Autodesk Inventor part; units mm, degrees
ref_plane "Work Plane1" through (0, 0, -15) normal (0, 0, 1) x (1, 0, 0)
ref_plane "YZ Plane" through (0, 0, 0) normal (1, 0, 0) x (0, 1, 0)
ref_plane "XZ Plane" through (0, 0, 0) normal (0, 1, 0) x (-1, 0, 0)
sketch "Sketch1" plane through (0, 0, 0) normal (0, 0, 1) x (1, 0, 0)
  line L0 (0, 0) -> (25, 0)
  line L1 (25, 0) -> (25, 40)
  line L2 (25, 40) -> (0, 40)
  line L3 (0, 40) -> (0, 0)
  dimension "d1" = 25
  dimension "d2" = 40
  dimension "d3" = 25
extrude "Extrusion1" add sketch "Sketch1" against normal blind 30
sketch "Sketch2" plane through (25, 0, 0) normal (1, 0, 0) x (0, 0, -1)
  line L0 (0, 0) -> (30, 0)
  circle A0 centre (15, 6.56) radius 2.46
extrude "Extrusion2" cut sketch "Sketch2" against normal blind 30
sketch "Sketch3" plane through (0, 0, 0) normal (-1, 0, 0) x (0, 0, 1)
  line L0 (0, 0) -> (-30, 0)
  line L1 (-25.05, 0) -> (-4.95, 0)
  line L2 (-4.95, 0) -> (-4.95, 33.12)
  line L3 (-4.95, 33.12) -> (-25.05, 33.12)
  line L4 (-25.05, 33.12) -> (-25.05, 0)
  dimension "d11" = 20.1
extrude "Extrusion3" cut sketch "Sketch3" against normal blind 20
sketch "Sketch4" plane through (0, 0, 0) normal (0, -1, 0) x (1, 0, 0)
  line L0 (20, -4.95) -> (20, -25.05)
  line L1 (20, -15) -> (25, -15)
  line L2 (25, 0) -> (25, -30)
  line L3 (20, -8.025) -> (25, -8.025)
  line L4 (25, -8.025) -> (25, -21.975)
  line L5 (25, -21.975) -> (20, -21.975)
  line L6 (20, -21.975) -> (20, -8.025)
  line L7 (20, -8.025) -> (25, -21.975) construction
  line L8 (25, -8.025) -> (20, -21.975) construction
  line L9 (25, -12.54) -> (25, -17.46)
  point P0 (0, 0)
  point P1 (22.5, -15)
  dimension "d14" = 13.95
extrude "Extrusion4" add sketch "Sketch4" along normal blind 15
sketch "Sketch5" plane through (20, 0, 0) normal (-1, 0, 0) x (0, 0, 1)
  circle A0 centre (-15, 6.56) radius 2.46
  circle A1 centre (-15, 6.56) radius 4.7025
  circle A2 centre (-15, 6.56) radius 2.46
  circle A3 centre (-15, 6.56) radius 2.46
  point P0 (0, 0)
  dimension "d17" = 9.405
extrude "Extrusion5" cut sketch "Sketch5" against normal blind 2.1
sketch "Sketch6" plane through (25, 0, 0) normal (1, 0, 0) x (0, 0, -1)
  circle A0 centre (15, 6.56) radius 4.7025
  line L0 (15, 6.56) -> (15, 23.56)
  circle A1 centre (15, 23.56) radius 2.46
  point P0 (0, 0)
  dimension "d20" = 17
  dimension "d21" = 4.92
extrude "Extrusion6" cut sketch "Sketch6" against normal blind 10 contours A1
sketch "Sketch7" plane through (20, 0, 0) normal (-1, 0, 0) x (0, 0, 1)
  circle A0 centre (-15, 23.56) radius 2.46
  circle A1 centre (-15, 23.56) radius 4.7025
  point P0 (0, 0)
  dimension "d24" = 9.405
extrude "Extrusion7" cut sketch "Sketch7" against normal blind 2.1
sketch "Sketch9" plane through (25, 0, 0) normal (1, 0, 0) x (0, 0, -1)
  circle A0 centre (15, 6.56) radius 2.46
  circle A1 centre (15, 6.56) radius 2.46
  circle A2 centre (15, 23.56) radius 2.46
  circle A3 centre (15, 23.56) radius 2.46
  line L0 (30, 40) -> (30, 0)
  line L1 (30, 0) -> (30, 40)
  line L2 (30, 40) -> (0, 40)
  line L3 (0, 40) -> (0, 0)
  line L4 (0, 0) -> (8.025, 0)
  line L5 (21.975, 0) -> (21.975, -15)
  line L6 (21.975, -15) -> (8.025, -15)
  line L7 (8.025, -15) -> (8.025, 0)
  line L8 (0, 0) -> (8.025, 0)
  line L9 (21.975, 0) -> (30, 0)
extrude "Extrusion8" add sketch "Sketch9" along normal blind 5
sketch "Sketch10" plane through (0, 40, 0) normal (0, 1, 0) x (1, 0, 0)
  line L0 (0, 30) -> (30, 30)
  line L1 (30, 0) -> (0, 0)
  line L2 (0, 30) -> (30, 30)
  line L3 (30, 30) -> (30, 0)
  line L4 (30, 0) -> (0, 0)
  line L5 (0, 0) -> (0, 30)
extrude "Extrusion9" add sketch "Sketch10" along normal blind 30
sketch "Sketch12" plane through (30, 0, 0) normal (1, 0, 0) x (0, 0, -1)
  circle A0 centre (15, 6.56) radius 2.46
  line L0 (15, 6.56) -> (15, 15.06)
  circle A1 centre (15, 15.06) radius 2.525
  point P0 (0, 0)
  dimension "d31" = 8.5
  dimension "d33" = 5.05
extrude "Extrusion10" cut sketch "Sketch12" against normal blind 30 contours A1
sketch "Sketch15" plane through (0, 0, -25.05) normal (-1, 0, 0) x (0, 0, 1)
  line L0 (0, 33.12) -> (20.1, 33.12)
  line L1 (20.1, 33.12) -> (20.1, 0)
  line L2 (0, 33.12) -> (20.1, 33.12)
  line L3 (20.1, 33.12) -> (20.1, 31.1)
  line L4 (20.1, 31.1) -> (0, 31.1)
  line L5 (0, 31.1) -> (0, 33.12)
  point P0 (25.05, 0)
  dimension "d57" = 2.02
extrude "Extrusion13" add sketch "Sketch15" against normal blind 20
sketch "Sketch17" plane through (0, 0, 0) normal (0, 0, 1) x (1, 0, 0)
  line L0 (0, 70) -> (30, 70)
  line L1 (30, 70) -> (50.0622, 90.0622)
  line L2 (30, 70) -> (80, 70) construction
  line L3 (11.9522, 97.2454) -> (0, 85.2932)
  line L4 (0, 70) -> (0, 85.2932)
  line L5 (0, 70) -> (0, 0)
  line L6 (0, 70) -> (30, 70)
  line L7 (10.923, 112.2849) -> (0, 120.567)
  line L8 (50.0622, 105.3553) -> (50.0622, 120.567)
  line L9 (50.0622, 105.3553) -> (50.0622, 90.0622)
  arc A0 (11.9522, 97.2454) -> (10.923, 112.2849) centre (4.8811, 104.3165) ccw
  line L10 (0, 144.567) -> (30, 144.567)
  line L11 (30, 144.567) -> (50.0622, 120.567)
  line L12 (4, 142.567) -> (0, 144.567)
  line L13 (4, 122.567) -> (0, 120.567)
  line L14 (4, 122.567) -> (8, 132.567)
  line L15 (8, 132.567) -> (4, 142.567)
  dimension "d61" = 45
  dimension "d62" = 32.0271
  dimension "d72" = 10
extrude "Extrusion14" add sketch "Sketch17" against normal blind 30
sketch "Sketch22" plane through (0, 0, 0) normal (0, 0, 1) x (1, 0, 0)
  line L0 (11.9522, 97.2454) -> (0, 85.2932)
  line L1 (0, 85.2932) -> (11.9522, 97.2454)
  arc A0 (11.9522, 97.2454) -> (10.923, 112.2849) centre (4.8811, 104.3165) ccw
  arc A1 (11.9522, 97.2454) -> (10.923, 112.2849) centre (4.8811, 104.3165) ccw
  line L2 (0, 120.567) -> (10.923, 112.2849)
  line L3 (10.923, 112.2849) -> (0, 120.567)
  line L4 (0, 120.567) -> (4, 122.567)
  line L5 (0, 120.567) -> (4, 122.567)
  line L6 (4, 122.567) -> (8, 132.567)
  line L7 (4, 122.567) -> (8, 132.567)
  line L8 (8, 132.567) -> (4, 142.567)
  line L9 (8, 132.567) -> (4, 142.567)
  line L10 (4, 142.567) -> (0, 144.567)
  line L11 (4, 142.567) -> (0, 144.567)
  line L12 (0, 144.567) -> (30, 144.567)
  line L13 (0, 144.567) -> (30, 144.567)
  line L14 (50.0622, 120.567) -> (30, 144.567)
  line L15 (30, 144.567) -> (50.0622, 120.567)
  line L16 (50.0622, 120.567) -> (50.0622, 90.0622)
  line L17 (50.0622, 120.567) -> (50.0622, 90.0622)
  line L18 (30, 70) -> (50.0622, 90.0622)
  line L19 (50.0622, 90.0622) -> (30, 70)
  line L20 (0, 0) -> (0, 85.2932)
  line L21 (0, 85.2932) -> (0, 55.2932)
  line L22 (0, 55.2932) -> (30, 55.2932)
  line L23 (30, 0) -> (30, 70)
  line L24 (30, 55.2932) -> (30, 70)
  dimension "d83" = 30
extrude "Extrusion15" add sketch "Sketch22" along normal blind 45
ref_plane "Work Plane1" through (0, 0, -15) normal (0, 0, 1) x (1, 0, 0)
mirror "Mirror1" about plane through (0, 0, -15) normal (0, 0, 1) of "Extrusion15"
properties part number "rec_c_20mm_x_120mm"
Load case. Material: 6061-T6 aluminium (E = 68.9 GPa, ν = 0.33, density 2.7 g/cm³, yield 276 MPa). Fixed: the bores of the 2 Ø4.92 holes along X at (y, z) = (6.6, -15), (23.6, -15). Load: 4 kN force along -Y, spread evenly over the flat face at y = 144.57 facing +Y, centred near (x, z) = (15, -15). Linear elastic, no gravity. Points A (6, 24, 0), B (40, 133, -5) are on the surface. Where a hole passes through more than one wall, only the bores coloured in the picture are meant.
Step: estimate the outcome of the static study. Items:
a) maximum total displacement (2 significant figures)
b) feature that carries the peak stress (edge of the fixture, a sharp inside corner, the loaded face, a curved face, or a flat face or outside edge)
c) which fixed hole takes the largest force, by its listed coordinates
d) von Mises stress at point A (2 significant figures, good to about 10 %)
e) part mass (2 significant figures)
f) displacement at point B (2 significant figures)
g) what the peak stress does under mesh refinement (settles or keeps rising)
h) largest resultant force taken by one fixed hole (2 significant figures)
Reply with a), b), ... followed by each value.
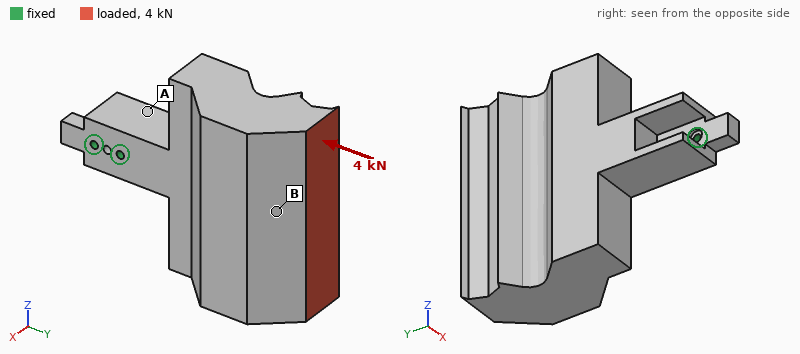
a) 0.12 mm
b) edge of the fixture
c) (23.6, -15)
d) 11 MPa
e) 1.2 kg
f) 0.10 mm
g) keeps rising
h) 3.0 kN
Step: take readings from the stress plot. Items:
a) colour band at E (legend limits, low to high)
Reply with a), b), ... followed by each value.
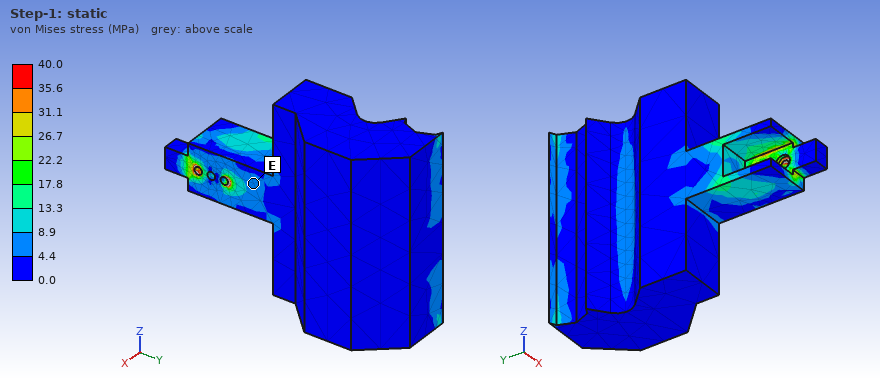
a) 4.4 to 8.9 MPa
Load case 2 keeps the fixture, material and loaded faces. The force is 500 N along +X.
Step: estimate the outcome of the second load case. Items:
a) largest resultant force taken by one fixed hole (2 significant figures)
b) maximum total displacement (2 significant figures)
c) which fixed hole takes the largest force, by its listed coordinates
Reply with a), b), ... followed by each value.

a) 2.9 kN
b) 0.21 mm
c) (23.6, -15)
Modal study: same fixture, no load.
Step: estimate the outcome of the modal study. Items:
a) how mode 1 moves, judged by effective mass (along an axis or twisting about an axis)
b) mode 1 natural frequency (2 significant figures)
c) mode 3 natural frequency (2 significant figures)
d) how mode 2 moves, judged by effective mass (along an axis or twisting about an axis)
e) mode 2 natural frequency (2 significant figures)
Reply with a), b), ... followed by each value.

a) along X
b) 360 Hz
c) 560 Hz
d) along Z
e) 380 Hz
